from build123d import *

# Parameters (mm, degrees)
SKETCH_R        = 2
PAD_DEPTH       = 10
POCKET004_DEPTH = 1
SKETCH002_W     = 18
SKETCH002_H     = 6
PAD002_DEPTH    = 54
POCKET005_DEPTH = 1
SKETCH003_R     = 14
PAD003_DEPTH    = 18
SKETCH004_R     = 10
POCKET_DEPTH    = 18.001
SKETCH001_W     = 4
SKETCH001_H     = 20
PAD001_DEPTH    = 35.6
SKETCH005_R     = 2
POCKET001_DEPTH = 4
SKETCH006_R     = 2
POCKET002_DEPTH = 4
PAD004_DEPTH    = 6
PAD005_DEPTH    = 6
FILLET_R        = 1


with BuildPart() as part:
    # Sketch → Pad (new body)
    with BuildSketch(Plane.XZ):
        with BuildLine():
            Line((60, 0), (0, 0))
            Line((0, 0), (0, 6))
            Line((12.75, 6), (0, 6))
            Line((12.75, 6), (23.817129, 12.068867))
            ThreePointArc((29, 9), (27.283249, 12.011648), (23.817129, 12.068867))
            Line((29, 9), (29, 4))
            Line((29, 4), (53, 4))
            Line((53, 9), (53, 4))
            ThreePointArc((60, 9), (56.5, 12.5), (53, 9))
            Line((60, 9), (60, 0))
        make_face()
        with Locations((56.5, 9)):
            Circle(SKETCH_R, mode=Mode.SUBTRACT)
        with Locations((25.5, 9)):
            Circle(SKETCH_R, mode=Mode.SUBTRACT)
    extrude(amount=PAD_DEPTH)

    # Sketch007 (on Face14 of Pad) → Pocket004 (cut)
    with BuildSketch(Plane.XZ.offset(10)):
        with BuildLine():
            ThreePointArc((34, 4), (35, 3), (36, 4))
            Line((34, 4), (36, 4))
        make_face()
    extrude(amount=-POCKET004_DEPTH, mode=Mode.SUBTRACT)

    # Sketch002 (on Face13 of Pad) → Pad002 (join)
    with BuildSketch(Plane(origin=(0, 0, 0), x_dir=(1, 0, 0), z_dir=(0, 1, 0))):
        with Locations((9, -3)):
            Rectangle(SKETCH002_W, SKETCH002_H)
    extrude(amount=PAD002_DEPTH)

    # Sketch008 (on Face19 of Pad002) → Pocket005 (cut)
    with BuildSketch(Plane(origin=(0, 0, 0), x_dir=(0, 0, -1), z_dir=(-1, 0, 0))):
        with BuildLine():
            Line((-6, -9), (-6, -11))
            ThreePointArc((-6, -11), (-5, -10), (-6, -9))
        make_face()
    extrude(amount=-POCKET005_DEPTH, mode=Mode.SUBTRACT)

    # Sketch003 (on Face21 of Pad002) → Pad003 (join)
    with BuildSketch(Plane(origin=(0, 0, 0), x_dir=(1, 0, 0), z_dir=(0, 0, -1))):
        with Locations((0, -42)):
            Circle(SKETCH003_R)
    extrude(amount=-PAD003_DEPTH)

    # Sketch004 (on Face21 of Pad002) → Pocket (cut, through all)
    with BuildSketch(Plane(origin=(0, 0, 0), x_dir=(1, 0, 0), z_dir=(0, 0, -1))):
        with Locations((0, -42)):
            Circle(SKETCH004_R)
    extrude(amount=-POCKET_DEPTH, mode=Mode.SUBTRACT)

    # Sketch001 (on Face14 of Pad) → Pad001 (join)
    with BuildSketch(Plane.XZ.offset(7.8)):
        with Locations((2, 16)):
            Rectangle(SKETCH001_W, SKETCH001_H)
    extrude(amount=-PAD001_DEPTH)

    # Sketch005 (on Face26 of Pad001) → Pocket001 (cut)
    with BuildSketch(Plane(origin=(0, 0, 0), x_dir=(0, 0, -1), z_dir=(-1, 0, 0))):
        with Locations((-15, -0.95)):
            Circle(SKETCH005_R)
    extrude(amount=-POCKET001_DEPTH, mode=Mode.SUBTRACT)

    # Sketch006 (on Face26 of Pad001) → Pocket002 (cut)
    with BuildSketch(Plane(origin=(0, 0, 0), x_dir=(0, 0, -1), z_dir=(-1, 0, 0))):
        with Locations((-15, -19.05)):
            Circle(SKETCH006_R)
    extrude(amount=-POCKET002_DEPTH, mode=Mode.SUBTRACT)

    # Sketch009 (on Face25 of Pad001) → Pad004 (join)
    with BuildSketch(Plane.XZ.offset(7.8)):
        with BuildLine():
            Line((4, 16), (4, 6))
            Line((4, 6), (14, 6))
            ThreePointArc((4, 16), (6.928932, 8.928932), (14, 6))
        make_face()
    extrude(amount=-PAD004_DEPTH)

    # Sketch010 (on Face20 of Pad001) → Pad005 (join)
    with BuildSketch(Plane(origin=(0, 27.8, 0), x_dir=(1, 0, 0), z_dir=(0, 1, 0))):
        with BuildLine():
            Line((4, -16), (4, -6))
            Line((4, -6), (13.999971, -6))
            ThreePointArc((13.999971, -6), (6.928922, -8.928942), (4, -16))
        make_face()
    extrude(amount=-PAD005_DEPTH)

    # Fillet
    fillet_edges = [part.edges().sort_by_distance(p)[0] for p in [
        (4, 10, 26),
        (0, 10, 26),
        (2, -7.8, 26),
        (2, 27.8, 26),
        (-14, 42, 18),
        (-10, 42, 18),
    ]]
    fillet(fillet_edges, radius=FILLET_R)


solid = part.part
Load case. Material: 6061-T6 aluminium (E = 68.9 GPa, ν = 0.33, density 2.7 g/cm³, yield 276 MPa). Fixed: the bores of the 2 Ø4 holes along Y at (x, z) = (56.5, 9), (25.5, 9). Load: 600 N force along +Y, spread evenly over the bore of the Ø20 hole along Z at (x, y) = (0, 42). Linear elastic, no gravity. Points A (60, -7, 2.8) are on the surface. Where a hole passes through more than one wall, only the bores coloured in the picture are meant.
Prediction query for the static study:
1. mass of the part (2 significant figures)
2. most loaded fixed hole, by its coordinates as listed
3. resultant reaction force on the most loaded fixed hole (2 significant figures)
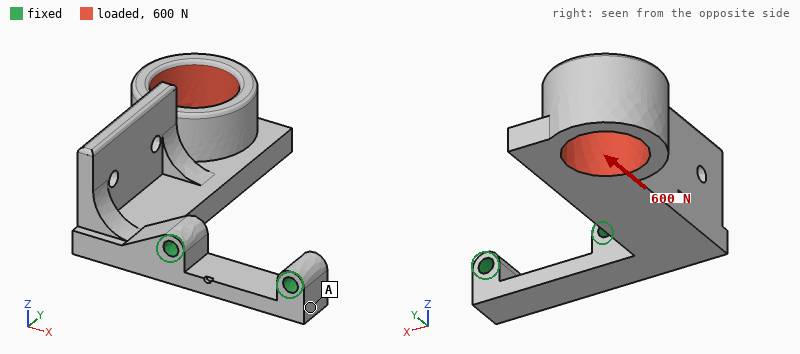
44 g
(25.5, 9)
680 N
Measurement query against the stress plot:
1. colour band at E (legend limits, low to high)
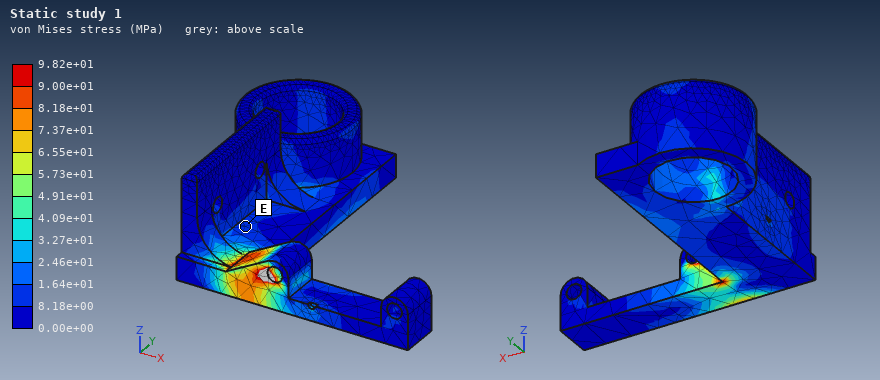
8.18e+00 to 1.64e+01 MPa
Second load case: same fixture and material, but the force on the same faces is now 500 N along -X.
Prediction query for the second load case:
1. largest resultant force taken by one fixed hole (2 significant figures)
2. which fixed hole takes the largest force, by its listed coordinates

500 N
(25.5, 9)
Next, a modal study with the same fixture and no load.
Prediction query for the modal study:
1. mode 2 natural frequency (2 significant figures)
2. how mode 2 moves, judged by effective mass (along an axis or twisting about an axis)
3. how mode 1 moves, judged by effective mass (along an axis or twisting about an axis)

1100 Hz
along X
along Z
